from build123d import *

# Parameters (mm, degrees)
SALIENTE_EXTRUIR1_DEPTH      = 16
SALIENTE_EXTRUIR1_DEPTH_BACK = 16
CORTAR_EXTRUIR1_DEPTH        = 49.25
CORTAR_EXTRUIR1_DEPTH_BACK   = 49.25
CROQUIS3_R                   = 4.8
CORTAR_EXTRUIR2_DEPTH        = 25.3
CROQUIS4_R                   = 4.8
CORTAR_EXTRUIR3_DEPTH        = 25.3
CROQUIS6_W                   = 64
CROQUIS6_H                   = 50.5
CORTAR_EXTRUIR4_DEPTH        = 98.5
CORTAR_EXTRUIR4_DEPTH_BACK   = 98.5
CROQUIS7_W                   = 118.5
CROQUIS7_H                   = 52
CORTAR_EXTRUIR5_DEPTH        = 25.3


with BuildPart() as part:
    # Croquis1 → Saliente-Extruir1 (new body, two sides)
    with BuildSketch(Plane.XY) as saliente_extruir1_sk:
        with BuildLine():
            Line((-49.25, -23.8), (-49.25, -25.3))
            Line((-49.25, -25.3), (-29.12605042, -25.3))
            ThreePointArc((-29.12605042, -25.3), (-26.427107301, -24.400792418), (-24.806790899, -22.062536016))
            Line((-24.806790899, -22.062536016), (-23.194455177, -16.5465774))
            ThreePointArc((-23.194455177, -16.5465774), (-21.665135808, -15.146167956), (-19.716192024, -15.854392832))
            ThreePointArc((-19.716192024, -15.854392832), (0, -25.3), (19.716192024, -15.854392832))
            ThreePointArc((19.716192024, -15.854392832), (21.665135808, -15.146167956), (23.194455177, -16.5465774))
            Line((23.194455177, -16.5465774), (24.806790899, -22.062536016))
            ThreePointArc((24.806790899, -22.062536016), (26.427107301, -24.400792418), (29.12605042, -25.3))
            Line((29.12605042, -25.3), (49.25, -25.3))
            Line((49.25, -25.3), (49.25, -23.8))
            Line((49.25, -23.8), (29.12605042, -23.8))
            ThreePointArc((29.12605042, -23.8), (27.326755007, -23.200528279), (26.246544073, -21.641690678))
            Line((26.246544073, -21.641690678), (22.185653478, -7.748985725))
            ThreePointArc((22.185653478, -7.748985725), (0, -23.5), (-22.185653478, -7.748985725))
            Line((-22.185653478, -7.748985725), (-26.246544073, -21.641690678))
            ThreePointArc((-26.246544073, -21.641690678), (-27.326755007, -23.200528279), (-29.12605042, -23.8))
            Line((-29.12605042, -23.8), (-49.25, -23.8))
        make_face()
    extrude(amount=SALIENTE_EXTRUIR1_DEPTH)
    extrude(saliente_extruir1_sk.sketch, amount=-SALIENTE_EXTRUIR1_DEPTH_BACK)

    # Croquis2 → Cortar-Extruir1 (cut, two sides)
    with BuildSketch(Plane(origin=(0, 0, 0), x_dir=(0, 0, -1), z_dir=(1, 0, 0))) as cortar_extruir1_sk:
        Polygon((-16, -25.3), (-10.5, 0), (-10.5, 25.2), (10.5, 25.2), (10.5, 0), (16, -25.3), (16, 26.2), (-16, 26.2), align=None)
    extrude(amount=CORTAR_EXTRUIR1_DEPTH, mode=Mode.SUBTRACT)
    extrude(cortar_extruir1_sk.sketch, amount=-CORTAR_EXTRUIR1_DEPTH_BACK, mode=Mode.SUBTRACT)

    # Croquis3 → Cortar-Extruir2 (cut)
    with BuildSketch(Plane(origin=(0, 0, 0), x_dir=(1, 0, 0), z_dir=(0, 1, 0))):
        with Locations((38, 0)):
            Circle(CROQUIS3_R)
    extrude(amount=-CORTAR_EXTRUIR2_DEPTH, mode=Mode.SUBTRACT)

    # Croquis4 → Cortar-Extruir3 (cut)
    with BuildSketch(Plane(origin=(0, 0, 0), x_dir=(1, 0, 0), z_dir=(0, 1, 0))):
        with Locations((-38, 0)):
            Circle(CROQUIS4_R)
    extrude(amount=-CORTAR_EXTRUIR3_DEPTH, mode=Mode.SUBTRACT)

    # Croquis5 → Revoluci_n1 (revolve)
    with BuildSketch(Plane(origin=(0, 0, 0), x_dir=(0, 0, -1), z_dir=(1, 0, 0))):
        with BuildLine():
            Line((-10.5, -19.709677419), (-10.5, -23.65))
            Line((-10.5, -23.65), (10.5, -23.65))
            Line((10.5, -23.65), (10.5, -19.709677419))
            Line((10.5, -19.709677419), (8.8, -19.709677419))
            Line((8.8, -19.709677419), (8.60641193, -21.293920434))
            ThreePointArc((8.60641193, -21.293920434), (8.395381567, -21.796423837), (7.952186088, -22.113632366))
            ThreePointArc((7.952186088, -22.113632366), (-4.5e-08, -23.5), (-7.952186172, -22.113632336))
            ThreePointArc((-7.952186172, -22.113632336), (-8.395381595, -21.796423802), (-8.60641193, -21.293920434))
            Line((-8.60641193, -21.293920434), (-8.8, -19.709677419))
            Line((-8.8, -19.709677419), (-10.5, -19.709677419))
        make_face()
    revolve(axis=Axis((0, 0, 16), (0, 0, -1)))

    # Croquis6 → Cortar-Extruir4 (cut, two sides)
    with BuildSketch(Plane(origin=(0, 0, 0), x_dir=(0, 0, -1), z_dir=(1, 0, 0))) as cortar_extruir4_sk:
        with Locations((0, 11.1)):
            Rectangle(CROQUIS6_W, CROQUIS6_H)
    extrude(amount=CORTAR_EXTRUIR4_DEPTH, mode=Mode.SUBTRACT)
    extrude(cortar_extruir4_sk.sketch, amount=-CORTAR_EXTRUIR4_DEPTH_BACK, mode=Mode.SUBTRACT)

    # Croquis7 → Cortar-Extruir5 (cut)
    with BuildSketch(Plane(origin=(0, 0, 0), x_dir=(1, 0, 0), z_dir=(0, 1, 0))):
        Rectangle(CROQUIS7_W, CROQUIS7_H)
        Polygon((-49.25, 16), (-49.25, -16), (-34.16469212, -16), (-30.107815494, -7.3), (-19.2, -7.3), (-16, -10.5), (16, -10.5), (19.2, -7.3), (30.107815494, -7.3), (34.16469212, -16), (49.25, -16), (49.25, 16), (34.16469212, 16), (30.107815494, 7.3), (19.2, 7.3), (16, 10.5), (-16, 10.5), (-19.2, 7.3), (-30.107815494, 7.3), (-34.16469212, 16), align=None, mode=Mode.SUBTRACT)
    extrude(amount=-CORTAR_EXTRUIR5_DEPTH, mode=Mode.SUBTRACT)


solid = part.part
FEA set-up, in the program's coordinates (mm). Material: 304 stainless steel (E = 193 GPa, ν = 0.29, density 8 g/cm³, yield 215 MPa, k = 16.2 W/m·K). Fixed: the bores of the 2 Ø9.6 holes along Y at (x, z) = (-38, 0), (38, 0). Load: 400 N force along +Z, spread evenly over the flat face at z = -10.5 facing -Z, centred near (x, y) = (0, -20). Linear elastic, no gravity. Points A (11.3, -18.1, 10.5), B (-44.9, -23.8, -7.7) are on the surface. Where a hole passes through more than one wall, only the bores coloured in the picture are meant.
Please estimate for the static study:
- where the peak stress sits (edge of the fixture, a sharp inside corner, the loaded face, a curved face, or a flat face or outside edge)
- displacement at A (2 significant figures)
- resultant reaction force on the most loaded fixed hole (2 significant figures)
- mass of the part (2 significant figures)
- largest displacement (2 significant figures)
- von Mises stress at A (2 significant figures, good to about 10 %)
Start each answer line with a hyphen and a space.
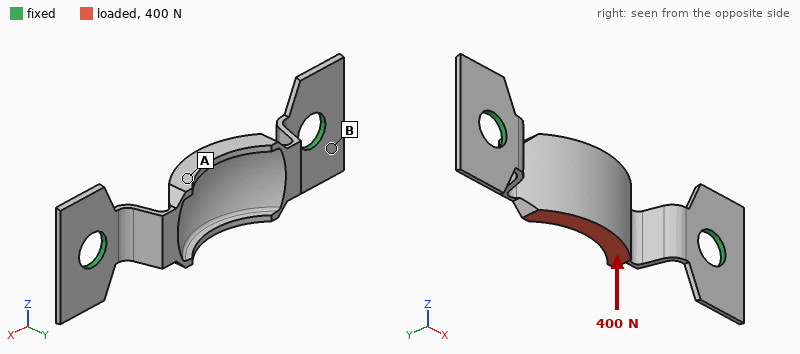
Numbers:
- a flat face or outside edge
- 39 µm
- 200 N
- 38 g
- 54 µm
- 27 MPa
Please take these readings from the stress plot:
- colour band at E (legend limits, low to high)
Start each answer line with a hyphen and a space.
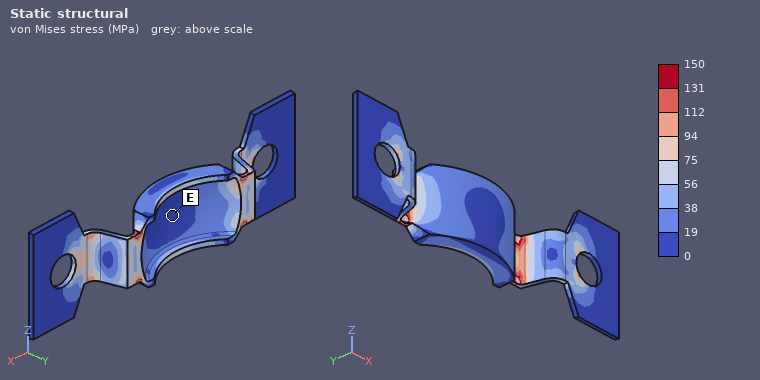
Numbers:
- 0 to 19 MPa
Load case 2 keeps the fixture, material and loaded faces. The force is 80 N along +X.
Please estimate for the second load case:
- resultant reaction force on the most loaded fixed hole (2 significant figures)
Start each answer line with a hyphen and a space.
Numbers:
- 43 N
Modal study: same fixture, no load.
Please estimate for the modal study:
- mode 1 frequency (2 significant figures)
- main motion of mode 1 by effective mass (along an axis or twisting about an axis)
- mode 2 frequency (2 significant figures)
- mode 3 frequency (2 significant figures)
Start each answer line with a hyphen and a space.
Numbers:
- 1800 Hz
- along X
- 2500 Hz
- 2600 Hz
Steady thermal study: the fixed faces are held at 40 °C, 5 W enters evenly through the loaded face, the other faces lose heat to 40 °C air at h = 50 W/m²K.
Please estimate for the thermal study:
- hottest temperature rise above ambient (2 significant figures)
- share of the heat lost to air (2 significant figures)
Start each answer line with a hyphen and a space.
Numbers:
- 59 K
- 89 %
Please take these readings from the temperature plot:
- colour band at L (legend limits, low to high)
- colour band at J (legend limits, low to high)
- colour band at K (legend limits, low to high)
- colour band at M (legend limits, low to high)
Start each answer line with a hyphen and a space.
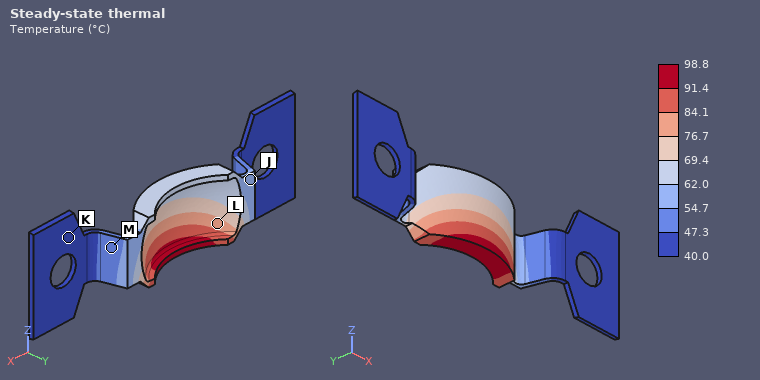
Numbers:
- 76.7 to 84.1 °C
- 54.7 to 62.0 °C
- 40.0 to 47.3 °C
- 47.3 to 54.7 °C
